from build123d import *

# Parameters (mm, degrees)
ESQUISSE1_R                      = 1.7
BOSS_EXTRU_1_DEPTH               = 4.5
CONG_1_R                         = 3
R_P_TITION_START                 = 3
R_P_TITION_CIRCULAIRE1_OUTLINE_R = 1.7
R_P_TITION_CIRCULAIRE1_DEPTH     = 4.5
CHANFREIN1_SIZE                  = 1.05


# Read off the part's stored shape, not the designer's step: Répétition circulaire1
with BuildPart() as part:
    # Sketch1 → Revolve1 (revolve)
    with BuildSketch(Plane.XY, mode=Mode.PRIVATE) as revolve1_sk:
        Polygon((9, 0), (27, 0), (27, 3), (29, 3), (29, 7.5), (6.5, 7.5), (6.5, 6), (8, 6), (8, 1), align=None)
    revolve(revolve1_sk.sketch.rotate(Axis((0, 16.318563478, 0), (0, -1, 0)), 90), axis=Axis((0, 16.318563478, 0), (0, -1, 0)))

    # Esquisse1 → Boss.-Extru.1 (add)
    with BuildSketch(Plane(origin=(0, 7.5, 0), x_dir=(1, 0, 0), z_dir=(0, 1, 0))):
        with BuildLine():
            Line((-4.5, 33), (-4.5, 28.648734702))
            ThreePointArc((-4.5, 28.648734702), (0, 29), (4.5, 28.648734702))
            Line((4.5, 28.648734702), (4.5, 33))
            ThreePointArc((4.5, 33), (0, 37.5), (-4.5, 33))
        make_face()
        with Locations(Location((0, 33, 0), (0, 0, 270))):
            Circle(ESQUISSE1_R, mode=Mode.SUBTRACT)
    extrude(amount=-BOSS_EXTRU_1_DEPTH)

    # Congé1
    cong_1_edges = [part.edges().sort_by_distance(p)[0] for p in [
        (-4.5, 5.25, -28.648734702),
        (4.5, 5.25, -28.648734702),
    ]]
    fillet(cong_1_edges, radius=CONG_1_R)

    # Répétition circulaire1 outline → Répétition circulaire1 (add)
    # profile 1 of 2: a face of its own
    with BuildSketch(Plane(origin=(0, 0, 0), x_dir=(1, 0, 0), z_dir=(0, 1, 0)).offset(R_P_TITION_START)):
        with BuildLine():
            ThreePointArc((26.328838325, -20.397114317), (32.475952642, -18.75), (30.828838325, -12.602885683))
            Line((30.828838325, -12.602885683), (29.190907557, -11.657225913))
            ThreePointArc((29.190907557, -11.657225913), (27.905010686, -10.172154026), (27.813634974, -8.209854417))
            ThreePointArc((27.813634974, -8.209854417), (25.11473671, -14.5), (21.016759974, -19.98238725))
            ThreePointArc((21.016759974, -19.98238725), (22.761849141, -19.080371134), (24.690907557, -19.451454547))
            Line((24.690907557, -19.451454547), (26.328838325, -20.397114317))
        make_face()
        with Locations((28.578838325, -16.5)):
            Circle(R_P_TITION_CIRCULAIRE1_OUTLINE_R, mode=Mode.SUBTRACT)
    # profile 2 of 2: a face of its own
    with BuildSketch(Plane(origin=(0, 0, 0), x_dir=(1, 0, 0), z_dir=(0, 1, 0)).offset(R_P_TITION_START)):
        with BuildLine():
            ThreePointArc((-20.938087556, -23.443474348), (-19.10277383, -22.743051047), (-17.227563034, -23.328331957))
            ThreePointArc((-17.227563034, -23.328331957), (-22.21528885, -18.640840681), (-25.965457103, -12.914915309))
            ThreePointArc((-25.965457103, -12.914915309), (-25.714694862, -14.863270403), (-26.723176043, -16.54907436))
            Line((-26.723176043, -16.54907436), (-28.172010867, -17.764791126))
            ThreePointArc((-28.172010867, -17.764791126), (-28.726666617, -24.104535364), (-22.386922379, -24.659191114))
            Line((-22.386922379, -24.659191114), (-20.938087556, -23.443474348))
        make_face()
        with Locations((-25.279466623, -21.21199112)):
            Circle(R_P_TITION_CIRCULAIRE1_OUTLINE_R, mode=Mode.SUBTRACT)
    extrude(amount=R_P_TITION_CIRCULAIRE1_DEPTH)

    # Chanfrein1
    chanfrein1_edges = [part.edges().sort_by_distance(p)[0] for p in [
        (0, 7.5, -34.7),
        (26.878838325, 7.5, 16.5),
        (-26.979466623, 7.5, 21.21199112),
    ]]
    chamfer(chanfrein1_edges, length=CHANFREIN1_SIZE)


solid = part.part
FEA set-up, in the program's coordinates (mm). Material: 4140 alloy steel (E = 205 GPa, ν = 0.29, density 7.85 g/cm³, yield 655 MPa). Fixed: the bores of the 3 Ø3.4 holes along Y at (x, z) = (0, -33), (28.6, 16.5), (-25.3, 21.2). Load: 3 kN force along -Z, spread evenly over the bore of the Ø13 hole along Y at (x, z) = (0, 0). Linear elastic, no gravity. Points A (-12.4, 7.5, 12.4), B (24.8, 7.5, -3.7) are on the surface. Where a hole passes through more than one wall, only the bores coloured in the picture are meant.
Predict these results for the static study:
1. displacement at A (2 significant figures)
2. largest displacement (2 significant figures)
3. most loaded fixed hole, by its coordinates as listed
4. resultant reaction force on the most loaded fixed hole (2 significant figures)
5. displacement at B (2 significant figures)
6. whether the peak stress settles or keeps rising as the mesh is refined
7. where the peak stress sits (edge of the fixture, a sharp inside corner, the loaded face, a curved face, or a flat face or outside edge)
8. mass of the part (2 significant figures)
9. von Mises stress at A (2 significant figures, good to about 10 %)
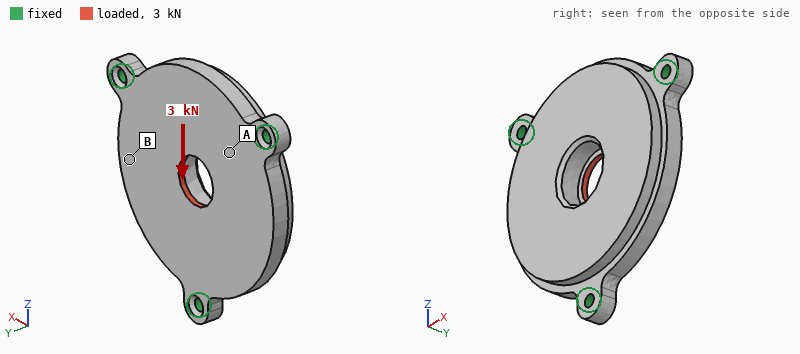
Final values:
2.7 µm
4.8 µm
(0, -33)
1.3 kN
2.4 µm
keeps rising
edge of the fixture
140 g
16 MPa
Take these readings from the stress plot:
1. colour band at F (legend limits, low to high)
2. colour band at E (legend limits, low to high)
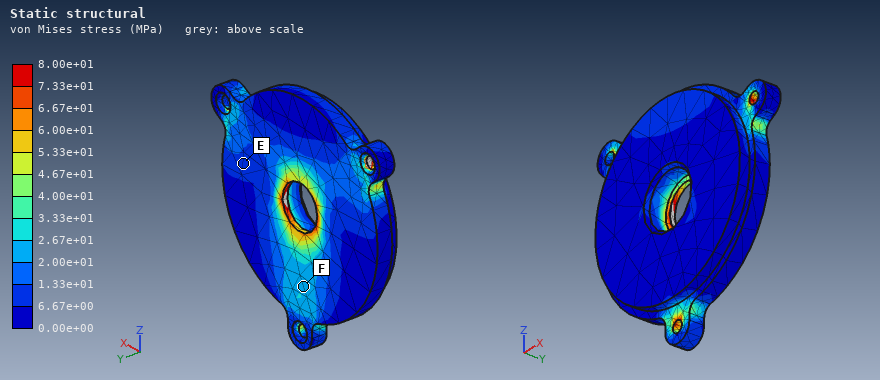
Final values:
2.00e+01 to 2.67e+01 MPa
6.67e+00 to 1.33e+01 MPa
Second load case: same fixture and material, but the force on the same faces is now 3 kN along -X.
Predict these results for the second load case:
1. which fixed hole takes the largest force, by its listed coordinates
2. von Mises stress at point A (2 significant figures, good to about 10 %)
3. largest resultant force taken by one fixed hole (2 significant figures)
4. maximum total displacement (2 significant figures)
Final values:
(28.6, 16.5)
20 MPa
1.2 kN
6.0 µm
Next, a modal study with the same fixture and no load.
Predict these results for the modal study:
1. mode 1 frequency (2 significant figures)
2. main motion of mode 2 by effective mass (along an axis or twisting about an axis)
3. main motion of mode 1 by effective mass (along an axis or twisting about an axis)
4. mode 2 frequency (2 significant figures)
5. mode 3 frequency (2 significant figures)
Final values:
5900 Hz
along Y
along Y
6900 Hz
8100 Hz
